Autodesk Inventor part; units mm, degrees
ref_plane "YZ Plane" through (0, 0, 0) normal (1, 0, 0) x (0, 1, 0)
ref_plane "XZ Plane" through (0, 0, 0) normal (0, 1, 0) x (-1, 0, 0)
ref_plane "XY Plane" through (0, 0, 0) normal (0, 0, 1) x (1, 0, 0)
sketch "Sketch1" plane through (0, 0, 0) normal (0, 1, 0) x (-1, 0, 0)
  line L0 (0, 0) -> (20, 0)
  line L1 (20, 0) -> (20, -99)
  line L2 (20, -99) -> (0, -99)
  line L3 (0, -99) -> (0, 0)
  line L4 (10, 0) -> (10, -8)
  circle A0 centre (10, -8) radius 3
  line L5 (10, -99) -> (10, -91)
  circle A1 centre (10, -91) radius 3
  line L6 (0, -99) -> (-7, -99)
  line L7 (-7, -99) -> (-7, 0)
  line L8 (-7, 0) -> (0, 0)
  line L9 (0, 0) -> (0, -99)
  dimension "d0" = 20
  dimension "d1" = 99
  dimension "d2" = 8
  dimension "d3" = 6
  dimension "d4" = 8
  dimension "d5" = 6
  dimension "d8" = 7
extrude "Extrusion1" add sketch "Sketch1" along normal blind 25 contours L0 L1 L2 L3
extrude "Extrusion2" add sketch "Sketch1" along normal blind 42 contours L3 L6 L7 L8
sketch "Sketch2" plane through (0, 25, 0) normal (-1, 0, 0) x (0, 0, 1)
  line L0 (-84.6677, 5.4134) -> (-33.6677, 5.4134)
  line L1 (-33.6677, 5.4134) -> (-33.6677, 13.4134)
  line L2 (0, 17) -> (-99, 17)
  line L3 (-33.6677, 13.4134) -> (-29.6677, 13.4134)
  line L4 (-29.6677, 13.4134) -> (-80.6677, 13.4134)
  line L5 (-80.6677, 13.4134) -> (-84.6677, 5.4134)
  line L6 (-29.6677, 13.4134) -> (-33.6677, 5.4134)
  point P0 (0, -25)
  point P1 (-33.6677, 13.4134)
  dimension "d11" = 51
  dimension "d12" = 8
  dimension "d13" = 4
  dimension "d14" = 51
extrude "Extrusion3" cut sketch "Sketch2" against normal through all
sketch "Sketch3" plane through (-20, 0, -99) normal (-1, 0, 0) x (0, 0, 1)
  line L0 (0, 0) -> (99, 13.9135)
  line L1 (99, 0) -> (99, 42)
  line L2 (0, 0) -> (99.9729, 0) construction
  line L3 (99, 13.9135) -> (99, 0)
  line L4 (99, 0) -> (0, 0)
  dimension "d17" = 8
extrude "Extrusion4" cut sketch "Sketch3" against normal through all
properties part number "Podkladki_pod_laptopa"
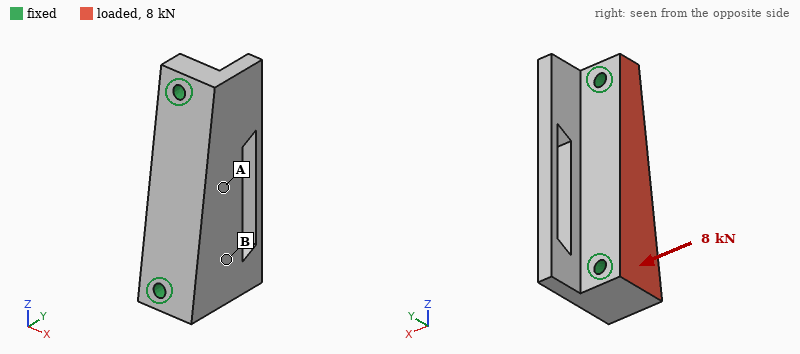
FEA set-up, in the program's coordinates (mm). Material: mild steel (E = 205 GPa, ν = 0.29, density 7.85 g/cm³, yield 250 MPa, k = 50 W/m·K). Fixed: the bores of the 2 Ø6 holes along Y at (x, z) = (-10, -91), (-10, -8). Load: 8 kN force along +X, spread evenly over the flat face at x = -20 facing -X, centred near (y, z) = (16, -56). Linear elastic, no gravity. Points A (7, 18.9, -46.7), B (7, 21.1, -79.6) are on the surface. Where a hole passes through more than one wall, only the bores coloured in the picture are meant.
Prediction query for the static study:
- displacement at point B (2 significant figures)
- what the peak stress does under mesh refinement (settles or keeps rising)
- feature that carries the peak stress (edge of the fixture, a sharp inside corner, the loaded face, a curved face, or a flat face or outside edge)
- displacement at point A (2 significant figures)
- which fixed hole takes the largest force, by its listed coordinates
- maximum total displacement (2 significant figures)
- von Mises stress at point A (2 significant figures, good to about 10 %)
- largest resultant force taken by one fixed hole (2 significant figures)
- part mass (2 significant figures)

2.9 µm
keeps rising
edge of the fixture
5.5 µm
(-10, -91)
5.9 µm
19 MPa
4.8 kN
440 g
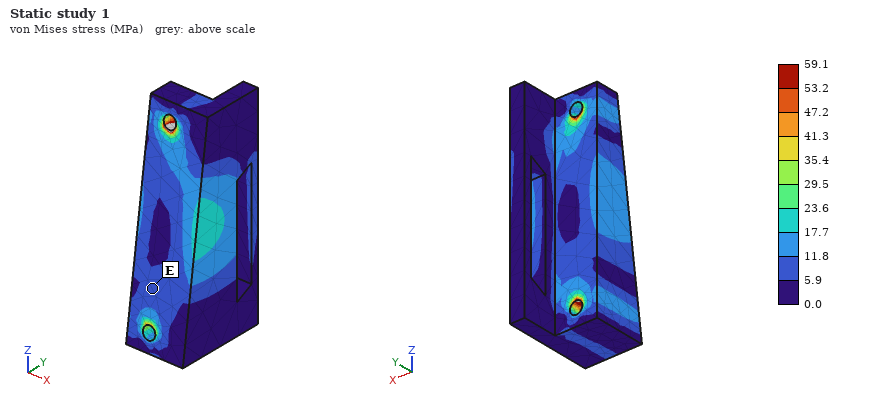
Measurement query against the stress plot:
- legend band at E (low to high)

5.9 to 11.8 MPa
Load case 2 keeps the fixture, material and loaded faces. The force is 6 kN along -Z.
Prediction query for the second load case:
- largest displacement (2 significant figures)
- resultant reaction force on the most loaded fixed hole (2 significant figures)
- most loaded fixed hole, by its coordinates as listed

1.4 µm
3.9 kN
(-10, -91)
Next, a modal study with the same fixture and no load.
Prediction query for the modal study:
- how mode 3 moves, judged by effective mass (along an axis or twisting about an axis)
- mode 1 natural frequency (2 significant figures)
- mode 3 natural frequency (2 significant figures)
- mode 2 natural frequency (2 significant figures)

along Y
6000 Hz
9300 Hz
6800 Hz
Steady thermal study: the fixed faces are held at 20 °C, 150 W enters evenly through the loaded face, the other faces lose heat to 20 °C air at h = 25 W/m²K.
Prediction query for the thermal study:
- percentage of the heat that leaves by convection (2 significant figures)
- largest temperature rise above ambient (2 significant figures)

5.1 %
68 K
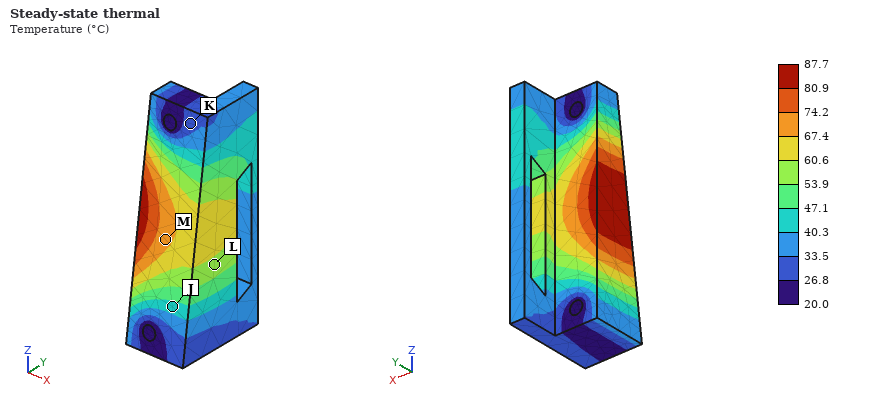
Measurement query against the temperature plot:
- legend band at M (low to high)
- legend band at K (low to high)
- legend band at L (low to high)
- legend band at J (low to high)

67.4 to 74.2 °C
26.8 to 33.5 °C
53.9 to 60.6 °C
40.3 to 47.1 °C
